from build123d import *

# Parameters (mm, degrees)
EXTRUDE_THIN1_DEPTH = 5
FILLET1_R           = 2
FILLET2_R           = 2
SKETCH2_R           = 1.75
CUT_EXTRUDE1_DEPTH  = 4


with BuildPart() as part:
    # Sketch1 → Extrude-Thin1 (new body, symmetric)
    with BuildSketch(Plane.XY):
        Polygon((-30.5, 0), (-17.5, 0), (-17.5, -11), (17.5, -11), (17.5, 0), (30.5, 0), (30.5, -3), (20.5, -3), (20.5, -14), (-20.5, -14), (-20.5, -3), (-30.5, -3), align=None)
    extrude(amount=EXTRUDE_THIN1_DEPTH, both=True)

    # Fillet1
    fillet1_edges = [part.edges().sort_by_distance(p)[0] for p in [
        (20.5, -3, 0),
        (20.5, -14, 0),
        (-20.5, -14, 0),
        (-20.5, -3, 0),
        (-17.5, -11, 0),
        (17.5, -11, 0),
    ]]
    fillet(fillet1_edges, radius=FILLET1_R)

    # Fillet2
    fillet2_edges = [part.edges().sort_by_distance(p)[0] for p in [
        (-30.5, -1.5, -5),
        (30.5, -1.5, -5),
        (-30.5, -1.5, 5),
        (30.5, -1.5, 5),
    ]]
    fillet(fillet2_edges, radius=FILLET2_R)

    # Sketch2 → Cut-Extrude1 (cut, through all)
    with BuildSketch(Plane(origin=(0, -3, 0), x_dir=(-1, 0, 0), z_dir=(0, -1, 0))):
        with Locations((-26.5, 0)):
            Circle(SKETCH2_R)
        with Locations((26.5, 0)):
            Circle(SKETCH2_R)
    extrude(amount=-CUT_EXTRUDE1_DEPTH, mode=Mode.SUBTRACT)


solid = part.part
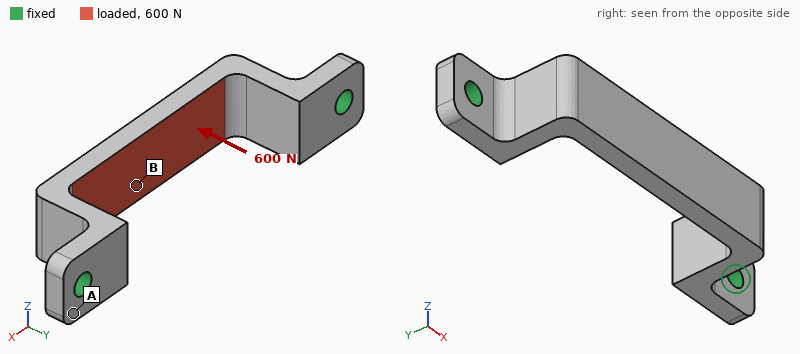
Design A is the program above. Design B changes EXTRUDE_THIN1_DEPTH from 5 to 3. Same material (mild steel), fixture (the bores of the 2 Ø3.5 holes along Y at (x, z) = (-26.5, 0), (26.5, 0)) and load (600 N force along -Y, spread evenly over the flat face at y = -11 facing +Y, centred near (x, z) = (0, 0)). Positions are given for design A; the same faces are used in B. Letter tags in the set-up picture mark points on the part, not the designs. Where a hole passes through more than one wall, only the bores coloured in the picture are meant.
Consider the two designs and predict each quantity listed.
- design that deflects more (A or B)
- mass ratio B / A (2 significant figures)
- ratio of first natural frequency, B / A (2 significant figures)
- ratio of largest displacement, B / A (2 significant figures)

B
0.59
0.86
1.6
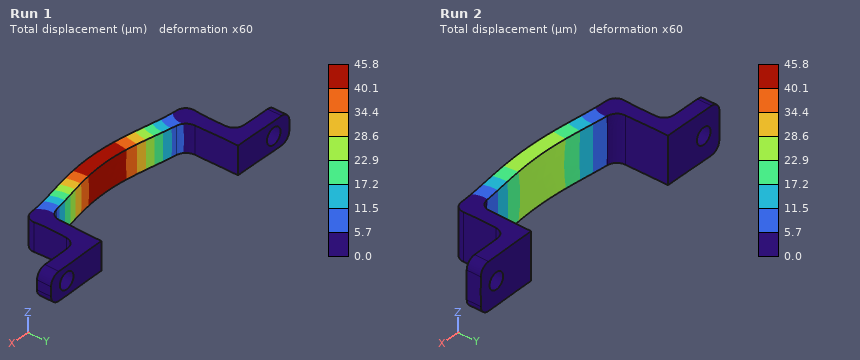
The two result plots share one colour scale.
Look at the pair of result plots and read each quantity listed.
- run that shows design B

Run 1
